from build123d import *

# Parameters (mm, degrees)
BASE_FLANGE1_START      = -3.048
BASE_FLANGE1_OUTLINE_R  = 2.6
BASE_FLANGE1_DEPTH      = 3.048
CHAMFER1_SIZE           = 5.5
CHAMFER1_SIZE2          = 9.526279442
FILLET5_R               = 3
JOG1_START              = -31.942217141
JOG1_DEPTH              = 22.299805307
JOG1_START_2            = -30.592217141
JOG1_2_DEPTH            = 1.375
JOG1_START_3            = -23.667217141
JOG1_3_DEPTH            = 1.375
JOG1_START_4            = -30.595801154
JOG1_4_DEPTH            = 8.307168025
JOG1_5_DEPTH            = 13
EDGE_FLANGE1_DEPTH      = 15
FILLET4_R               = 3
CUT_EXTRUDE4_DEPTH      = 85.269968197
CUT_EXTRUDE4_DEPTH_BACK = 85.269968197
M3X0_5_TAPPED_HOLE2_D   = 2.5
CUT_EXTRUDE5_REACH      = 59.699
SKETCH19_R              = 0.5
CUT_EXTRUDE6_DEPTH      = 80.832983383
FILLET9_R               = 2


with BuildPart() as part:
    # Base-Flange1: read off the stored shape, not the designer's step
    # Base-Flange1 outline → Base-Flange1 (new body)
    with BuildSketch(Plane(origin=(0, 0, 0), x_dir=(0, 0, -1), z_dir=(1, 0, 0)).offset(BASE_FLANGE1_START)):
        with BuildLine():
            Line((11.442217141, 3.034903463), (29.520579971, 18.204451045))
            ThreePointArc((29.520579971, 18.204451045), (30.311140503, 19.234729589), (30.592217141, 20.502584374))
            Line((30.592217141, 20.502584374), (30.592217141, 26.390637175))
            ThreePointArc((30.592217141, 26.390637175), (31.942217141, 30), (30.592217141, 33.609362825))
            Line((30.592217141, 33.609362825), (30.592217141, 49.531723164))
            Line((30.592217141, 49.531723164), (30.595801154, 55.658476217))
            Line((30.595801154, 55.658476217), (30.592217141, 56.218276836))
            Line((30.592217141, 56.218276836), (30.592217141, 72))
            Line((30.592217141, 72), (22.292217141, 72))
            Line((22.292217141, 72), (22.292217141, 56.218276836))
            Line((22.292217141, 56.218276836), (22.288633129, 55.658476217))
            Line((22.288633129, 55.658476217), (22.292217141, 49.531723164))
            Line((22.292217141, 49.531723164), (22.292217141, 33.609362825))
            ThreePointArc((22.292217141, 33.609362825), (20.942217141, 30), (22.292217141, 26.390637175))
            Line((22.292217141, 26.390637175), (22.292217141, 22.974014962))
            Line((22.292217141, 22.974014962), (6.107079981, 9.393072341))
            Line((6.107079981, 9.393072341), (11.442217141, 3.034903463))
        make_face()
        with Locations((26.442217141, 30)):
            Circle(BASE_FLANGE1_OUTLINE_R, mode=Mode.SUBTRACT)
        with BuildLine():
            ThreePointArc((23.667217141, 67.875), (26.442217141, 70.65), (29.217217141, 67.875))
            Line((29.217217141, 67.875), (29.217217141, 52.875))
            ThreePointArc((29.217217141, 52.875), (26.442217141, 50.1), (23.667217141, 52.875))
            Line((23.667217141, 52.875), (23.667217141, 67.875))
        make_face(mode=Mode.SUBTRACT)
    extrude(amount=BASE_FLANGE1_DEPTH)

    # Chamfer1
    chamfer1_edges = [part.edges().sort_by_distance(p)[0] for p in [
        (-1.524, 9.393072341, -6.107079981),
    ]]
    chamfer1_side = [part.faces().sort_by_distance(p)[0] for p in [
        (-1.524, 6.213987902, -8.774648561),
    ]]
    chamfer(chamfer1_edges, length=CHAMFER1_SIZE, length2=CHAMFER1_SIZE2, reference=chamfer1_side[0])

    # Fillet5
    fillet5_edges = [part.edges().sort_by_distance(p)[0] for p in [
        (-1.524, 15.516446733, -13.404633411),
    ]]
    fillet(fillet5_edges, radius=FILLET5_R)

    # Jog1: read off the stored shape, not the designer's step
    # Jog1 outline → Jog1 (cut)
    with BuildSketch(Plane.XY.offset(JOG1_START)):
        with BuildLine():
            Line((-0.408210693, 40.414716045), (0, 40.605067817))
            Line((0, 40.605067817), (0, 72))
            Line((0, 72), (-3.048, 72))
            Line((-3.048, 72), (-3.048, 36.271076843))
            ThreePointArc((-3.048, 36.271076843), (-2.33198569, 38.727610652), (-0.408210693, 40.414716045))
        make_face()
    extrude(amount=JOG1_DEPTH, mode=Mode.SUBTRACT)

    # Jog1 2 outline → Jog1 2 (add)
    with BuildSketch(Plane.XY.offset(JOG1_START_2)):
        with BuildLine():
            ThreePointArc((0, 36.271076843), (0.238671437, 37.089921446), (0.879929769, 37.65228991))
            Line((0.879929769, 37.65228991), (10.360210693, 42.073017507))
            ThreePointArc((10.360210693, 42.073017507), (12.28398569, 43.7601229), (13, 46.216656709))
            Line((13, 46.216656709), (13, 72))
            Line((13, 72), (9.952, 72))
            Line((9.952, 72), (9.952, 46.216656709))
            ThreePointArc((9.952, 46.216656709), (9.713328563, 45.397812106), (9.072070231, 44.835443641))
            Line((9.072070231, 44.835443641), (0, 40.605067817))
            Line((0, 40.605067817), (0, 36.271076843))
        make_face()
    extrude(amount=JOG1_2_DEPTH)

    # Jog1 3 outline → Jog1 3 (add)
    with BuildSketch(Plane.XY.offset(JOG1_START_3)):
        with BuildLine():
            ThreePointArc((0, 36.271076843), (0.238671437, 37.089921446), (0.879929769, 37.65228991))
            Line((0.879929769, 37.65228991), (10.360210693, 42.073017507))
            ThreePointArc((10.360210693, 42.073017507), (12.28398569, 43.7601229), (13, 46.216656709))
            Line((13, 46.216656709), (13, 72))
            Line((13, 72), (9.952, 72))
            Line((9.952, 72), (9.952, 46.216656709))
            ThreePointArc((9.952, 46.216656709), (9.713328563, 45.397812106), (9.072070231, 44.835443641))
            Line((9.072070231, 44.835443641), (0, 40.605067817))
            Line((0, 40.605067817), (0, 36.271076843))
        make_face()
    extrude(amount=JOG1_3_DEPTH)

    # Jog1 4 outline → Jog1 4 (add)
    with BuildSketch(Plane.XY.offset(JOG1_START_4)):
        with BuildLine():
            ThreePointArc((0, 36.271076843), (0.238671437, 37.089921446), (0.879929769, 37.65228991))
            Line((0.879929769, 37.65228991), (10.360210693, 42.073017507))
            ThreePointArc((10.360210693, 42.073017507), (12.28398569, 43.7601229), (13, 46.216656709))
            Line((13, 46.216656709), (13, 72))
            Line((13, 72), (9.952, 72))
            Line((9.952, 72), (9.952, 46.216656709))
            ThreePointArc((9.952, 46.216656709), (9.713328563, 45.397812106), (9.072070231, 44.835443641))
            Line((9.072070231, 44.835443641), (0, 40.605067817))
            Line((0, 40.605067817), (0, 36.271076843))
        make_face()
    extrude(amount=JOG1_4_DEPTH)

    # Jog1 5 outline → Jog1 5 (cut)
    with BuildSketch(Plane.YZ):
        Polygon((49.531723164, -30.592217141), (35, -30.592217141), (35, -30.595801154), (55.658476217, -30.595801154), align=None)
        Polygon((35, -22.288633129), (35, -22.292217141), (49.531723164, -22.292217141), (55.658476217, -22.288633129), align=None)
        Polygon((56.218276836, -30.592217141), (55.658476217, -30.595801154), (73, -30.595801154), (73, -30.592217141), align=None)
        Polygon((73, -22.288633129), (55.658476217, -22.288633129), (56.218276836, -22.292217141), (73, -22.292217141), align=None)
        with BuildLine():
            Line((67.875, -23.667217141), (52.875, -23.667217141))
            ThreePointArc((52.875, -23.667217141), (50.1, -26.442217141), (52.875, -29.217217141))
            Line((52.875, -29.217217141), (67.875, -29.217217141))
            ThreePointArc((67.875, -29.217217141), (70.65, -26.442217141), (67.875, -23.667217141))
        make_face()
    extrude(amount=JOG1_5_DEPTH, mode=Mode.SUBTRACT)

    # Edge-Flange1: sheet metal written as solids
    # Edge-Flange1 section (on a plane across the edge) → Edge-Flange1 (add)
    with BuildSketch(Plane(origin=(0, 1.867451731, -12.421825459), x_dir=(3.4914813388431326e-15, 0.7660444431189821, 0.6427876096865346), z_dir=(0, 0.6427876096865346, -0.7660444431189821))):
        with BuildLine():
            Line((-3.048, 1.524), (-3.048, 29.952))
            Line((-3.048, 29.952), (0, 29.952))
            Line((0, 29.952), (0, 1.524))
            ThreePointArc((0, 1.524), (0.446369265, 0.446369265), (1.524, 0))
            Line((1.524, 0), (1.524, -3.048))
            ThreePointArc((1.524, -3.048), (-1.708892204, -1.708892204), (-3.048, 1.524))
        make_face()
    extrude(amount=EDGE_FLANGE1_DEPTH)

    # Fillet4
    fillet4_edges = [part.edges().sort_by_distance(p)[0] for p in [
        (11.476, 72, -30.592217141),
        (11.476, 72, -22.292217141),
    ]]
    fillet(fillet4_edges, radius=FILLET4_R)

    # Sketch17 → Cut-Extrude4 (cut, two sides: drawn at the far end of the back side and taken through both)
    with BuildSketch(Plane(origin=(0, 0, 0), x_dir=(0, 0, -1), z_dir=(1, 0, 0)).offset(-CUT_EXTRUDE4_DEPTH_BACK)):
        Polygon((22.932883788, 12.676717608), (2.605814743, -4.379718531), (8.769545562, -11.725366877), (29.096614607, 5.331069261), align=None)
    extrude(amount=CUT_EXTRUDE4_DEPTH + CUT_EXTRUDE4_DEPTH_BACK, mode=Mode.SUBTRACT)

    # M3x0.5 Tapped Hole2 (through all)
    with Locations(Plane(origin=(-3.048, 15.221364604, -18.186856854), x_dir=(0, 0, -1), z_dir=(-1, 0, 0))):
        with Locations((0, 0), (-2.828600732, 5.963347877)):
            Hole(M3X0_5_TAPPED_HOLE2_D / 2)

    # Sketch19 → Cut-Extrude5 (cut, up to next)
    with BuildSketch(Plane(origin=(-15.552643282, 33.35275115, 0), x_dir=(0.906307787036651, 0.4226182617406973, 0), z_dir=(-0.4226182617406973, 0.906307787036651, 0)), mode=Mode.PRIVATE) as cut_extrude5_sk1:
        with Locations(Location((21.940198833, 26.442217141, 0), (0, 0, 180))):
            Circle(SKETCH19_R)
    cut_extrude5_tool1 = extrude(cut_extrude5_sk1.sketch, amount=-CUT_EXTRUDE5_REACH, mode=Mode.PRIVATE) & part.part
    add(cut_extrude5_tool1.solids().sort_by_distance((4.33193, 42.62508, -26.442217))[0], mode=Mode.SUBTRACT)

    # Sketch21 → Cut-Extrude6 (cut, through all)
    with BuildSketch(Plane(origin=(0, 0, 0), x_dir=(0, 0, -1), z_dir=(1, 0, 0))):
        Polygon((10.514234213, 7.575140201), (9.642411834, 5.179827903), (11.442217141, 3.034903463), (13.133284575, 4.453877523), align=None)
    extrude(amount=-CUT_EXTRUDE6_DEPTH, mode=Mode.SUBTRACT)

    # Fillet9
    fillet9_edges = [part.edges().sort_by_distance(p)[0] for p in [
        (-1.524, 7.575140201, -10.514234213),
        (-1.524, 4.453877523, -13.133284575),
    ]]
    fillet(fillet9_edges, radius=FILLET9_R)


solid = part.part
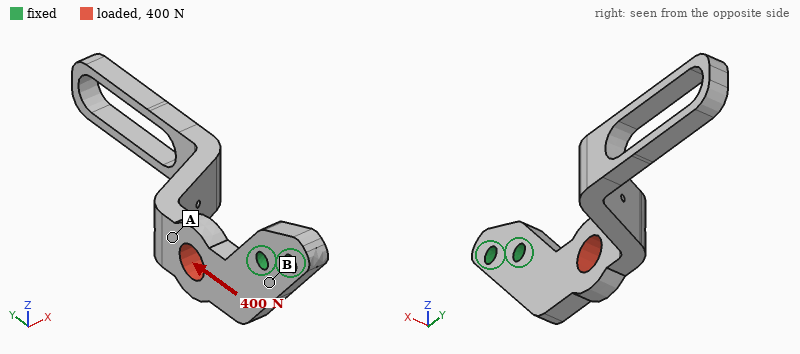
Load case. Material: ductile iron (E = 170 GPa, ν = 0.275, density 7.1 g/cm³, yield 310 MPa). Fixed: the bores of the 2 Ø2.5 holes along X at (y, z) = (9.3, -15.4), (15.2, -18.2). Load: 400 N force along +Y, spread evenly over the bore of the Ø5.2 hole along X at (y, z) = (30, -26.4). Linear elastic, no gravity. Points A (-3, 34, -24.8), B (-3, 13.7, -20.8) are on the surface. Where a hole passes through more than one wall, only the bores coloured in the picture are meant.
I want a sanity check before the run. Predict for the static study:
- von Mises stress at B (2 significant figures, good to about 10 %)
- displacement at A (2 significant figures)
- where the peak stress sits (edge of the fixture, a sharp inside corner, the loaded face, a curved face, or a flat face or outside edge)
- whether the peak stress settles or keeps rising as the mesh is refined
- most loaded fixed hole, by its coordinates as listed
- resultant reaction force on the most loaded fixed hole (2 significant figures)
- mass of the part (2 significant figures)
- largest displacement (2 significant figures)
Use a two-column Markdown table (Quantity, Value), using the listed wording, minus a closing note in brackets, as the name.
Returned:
| Quantity | Value |
|---|---|
| von Mises stress at B | 47 MPa |
| displacement at A | 19 µm |
| where the peak stress sits | edge of the fixture |
| whether the peak stress settles or keeps rising as the mesh is refined | keeps rising |
| most loaded fixed hole, by its coordinates as listed | (15.2, -18.2) |
| resultant reaction force on the most loaded fixed hole | 480 N |
| mass of the part | 11 g |
| largest displacement | 57 µm |
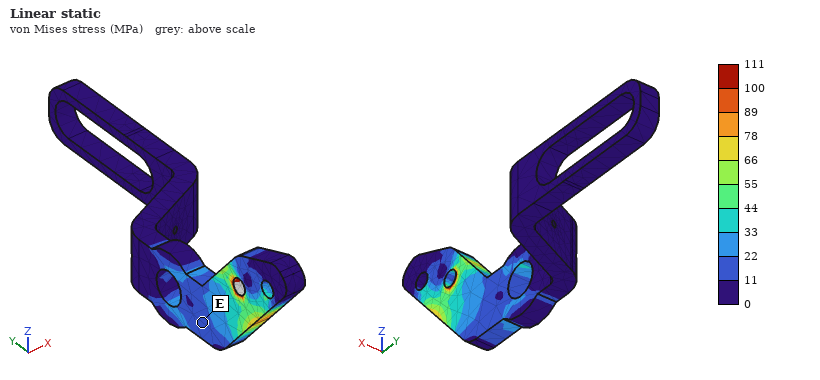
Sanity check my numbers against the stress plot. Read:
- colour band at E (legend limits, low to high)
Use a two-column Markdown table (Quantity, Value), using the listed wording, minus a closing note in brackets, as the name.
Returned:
| Quantity | Value |
|---|---|
| colour band at E | 11 to 22 MPa |
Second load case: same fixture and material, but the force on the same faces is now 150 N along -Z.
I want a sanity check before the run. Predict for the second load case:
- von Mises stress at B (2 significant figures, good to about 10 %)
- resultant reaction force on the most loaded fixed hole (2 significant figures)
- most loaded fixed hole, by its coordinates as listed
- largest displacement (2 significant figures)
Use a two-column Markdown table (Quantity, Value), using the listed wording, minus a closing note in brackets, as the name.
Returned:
| Quantity | Value |
|---|---|
| von Mises stress at B | 29 MPa |
| resultant reaction force on the most loaded fixed hole | 350 N |
| most loaded fixed hole, by its coordinates as listed | (15.2, -18.2) |
| largest displacement | 65 µm |
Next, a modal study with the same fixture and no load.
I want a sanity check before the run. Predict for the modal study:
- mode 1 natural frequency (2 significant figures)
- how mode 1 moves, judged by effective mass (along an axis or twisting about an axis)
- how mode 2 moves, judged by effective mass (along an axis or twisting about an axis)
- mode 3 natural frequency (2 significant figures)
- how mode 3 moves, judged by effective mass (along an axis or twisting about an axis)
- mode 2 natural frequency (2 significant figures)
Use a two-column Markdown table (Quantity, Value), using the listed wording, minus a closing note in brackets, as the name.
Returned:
| Quantity | Value |
|---|---|
| mode 1 natural frequency | 820 Hz |
| how mode 1 moves, judged by effective mass | along X |
| how mode 2 moves, judged by effective mass | along Z |
| mode 3 natural frequency | 3400 Hz |
| how mode 3 moves, judged by effective mass | along X |
| mode 2 natural frequency | 1600 Hz |
